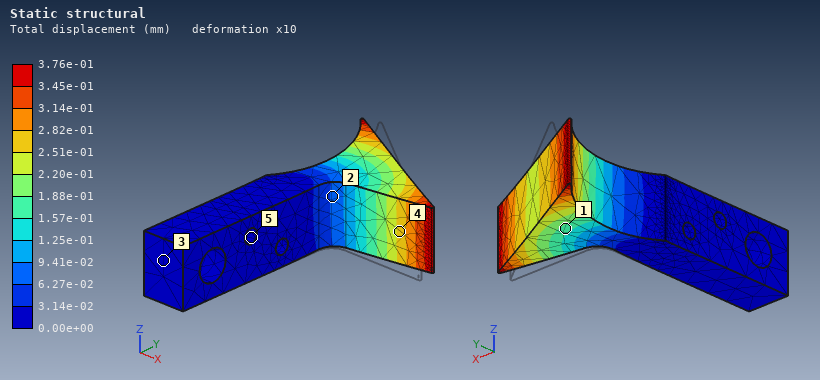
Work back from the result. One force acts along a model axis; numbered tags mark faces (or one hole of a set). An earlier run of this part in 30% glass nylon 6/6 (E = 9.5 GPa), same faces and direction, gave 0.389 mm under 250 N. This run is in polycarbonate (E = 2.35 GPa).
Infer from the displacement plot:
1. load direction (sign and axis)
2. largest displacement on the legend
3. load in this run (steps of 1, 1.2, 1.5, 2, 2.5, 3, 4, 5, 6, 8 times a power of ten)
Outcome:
+Y
3.76e-01 mm
60 N
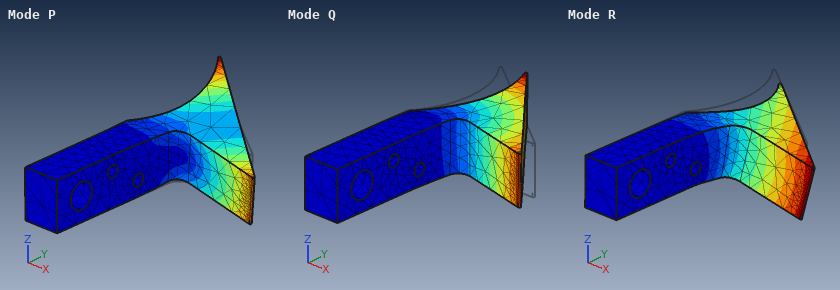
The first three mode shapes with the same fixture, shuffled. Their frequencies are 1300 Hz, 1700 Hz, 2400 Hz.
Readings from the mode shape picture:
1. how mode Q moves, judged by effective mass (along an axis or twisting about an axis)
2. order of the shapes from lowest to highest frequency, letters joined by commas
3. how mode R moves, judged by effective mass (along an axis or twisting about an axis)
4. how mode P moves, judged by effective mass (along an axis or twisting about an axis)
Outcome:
along X
Q, R, P
along Z
twisting about Y
